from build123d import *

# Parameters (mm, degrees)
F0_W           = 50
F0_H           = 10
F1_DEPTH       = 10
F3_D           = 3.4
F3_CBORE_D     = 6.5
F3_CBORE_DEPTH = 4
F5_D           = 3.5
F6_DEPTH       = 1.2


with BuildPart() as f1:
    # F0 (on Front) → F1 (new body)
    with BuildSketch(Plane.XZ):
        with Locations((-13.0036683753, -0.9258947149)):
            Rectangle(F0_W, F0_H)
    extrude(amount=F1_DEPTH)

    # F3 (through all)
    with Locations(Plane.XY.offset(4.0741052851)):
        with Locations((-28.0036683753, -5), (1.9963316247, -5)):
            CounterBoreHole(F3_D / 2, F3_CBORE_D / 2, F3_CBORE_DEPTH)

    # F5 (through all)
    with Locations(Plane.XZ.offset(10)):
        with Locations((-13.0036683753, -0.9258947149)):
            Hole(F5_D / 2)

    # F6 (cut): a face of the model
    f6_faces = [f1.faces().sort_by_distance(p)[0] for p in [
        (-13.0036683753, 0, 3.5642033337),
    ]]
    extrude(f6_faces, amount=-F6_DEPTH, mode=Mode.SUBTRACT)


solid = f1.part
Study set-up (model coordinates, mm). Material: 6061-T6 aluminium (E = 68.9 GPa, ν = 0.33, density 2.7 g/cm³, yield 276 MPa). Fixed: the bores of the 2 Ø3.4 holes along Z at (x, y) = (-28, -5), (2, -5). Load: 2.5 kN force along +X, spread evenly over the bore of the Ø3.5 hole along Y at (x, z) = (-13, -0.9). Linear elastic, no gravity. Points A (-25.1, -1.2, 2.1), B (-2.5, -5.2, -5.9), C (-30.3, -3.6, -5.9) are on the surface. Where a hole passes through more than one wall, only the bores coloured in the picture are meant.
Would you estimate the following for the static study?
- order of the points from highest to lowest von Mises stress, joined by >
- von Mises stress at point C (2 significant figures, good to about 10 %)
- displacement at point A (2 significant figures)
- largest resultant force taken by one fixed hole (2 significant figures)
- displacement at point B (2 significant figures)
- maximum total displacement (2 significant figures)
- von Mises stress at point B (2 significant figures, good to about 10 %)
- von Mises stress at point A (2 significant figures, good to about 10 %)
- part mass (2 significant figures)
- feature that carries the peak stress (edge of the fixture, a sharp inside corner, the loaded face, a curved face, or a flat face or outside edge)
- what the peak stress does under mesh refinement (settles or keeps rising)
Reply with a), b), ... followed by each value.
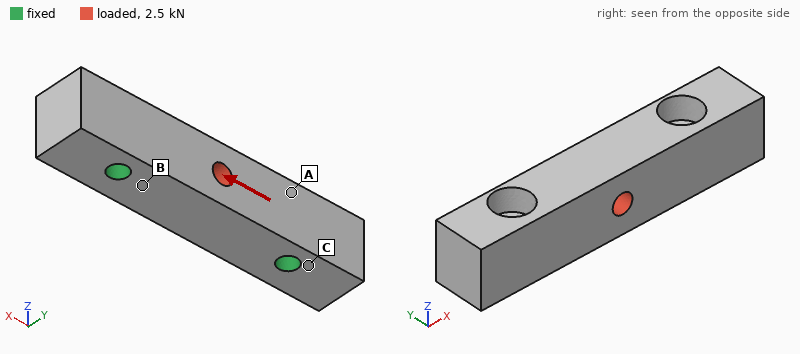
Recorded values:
a) B > A > C
b) 6.0 MPa
c) 1.9 µm
d) 1.3 kN
e) 1.1 µm
f) 4.6 µm
g) 23 MPa
h) 14 MPa
i) 11 g
j) edge of the fixture
k) keeps rising
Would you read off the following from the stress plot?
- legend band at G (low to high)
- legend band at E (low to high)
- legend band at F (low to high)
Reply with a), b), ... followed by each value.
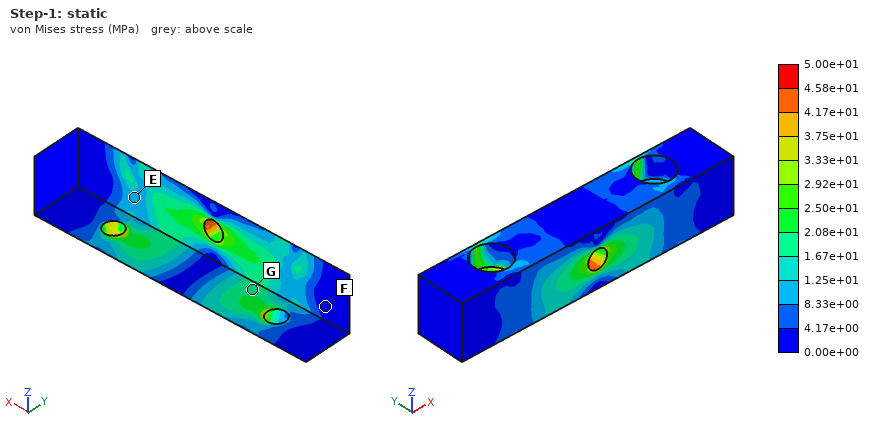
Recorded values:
a) 1.67e+01 to 2.08e+01 MPa
b) 8.33e+00 to 1.25e+01 MPa
c) 0.00e+00 to 4.17e+00 MPa
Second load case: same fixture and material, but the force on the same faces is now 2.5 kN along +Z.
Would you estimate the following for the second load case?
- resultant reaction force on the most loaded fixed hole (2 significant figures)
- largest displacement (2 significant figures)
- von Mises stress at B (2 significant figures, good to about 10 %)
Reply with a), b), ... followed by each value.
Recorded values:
a) 1.4 kN
b) 21 µm
c) 38 MPa
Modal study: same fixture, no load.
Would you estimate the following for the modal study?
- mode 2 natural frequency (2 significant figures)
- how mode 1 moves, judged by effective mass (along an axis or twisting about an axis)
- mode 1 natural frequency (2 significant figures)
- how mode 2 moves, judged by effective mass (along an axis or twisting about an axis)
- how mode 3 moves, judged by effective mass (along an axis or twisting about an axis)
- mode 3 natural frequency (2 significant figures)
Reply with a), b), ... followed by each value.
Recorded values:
a) 32 kHz
b) along Y
c) 26 kHz
d) along Z
e) along Y
f) 34 kHz
